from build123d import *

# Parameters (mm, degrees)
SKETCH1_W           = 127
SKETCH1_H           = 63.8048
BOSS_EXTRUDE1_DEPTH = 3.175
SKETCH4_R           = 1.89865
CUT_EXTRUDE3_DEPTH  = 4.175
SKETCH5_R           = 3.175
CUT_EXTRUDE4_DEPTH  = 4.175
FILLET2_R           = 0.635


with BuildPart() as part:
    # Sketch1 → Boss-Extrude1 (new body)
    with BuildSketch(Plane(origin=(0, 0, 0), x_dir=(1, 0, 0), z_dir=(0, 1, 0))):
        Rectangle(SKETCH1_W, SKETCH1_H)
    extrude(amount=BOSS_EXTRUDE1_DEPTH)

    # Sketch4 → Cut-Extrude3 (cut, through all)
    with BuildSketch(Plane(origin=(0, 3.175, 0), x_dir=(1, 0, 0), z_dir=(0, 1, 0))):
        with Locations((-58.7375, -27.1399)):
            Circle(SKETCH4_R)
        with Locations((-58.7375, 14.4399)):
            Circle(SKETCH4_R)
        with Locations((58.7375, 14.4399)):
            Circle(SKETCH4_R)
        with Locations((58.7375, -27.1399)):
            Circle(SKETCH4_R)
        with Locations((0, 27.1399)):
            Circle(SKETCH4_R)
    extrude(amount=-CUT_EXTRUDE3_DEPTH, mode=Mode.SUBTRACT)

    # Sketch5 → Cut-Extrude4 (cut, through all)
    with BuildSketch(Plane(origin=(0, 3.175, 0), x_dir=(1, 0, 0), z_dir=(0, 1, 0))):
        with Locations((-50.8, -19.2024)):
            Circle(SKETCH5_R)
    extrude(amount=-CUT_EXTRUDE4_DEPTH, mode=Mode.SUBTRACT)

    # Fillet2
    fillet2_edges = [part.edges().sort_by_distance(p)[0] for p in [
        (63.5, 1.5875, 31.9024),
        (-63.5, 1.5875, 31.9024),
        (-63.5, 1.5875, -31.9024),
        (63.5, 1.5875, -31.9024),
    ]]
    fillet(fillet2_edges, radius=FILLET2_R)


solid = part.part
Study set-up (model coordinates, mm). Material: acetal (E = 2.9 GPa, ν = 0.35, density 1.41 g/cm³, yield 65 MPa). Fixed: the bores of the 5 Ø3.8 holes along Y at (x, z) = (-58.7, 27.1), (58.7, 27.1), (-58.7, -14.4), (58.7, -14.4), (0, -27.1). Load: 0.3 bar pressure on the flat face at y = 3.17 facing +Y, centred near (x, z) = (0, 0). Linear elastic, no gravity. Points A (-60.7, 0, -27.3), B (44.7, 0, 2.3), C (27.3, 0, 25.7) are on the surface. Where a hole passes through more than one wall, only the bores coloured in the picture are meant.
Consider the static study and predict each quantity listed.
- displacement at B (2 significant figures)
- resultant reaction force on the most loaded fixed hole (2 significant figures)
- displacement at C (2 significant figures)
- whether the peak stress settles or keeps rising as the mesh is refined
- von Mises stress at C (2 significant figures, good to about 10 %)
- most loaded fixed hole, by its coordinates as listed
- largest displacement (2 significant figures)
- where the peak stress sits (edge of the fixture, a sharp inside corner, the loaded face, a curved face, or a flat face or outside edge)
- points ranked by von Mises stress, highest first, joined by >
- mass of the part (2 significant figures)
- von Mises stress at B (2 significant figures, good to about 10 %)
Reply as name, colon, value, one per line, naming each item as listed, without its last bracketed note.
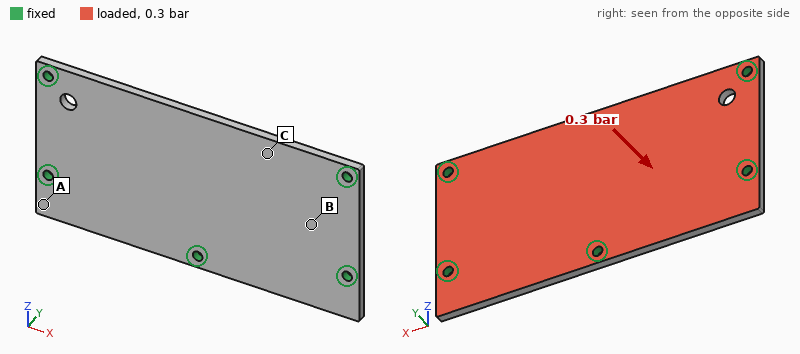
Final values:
displacement at B: 0.27 mm
resultant reaction force on the most loaded fixed hole: 81 N
displacement at C: 0.97 mm
whether the peak stress settles or keeps rising as the mesh is refined: keeps rising
von Mises stress at C: 6.4 MPa
most loaded fixed hole, by its coordinates as listed: (0, -27.1)
largest displacement: 1.7 mm
where the peak stress sits: edge of the fixture
points ranked by von Mises stress, highest first, joined by >: C > B > A
mass of the part: 36 g
von Mises stress at B: 3.4 MPa
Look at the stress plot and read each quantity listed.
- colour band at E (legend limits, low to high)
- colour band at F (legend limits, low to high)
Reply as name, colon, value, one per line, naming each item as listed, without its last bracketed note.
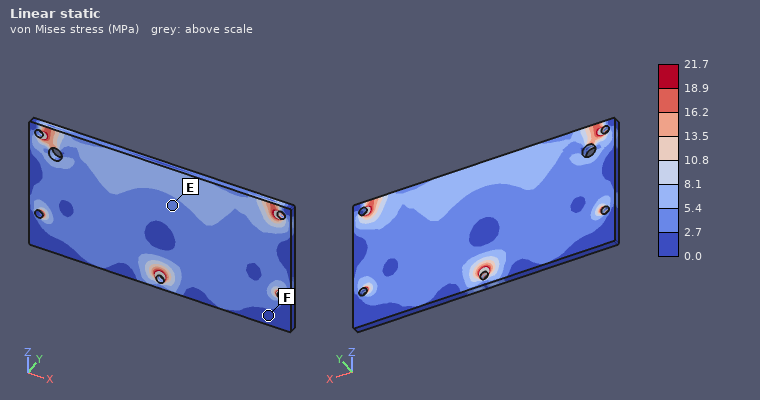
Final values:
colour band at E: 2.7 to 5.4 MPa
colour band at F: 0.0 to 2.7 MPa
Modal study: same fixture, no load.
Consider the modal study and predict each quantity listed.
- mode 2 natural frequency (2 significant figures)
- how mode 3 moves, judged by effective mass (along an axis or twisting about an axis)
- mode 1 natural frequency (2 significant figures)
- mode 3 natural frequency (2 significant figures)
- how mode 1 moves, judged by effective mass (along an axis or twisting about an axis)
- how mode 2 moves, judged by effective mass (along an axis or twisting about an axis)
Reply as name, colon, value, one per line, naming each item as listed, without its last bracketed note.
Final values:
mode 2 natural frequency: 940 Hz
how mode 3 moves, judged by effective mass: along Y
mode 1 natural frequency: 430 Hz
mode 3 natural frequency: 1200 Hz
how mode 1 moves, judged by effective mass: along Y
how mode 2 moves, judged by effective mass: twisting about Z
